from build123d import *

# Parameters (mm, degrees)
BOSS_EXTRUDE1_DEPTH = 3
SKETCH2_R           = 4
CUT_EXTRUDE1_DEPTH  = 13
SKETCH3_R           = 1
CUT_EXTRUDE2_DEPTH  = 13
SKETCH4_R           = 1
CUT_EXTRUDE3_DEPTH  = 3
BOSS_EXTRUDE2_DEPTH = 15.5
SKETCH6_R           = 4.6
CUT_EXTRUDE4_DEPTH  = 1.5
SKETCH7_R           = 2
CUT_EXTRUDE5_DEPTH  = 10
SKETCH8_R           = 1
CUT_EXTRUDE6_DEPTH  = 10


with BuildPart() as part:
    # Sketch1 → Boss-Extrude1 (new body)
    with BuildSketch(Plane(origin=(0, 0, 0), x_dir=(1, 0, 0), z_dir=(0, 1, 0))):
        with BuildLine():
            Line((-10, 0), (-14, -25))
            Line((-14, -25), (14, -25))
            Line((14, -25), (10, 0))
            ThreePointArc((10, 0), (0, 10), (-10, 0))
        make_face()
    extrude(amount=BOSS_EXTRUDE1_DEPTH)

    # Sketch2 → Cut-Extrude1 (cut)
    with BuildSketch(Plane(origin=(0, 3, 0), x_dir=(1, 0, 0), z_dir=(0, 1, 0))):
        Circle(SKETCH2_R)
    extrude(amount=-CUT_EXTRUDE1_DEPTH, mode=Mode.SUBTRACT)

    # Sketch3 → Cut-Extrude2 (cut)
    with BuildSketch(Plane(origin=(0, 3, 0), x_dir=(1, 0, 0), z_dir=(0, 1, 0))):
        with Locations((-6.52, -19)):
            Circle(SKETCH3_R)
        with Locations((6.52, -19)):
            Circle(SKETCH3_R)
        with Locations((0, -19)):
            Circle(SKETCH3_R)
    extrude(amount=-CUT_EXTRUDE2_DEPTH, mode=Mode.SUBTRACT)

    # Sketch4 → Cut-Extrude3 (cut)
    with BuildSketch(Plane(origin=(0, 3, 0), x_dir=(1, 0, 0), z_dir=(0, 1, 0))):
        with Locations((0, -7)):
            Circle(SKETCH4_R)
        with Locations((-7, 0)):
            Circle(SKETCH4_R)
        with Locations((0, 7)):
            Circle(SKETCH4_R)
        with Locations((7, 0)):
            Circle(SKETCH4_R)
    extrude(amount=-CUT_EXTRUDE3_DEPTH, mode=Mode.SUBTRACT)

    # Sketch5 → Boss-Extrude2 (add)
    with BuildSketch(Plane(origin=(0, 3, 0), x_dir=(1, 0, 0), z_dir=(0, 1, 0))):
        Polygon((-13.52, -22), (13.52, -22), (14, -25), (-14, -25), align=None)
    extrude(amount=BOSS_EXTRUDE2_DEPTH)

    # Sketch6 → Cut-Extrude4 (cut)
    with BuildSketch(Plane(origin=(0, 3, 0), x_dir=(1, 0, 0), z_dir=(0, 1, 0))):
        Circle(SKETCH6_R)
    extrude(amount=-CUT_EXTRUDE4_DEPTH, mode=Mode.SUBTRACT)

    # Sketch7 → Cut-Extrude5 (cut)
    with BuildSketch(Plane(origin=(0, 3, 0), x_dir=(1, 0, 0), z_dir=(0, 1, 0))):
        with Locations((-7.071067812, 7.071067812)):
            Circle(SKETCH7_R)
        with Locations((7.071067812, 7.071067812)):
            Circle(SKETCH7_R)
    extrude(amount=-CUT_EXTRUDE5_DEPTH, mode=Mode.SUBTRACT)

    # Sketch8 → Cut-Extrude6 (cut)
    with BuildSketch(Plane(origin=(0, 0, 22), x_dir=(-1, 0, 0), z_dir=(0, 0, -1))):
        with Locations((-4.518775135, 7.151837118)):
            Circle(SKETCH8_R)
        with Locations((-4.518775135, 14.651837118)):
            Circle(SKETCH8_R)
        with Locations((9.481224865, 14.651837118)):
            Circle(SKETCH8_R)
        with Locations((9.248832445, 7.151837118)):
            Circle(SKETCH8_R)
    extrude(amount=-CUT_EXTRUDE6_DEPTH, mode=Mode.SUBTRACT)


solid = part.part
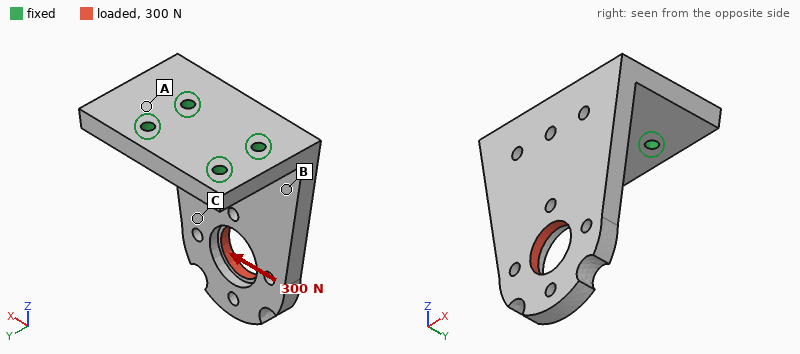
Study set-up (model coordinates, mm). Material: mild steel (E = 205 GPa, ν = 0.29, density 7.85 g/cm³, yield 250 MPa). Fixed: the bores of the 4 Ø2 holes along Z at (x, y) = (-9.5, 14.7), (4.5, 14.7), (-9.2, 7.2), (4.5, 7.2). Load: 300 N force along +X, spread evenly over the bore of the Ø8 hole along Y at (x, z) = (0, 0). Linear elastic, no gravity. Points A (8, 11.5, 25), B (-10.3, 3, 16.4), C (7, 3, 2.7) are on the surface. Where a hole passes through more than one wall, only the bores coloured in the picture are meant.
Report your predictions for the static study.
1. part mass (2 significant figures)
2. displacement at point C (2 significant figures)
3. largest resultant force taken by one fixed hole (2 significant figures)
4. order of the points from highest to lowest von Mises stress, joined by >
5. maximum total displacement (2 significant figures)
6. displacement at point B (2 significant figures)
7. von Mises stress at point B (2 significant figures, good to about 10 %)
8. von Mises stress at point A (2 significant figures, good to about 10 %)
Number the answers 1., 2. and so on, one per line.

1. 25 g
2. 16 µm
3. 500 N
4. B > A > C
5. 24 µm
6. 7.3 µm
7. 36 MPa
8. 26 MPa
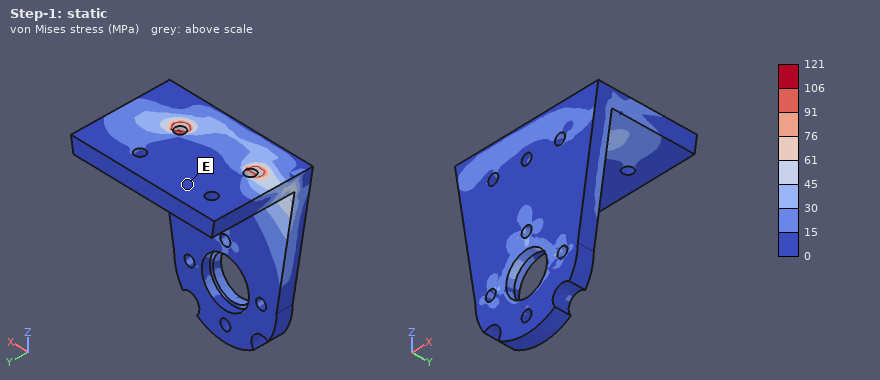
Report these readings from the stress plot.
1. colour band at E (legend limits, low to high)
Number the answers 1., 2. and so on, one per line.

1. 0 to 15 MPa
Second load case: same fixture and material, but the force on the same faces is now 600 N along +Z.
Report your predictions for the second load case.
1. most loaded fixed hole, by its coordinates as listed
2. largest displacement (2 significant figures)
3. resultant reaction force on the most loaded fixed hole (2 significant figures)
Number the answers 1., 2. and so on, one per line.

1. (4.5, 7.2)
2. 62 µm
3. 490 N
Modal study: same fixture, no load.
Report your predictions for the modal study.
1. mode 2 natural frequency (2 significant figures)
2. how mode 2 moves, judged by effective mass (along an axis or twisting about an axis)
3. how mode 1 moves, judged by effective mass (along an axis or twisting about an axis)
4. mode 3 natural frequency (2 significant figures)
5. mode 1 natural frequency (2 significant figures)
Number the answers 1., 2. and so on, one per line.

1. 7100 Hz
2. along X
3. along Y
4. 9700 Hz
5. 2400 Hz
